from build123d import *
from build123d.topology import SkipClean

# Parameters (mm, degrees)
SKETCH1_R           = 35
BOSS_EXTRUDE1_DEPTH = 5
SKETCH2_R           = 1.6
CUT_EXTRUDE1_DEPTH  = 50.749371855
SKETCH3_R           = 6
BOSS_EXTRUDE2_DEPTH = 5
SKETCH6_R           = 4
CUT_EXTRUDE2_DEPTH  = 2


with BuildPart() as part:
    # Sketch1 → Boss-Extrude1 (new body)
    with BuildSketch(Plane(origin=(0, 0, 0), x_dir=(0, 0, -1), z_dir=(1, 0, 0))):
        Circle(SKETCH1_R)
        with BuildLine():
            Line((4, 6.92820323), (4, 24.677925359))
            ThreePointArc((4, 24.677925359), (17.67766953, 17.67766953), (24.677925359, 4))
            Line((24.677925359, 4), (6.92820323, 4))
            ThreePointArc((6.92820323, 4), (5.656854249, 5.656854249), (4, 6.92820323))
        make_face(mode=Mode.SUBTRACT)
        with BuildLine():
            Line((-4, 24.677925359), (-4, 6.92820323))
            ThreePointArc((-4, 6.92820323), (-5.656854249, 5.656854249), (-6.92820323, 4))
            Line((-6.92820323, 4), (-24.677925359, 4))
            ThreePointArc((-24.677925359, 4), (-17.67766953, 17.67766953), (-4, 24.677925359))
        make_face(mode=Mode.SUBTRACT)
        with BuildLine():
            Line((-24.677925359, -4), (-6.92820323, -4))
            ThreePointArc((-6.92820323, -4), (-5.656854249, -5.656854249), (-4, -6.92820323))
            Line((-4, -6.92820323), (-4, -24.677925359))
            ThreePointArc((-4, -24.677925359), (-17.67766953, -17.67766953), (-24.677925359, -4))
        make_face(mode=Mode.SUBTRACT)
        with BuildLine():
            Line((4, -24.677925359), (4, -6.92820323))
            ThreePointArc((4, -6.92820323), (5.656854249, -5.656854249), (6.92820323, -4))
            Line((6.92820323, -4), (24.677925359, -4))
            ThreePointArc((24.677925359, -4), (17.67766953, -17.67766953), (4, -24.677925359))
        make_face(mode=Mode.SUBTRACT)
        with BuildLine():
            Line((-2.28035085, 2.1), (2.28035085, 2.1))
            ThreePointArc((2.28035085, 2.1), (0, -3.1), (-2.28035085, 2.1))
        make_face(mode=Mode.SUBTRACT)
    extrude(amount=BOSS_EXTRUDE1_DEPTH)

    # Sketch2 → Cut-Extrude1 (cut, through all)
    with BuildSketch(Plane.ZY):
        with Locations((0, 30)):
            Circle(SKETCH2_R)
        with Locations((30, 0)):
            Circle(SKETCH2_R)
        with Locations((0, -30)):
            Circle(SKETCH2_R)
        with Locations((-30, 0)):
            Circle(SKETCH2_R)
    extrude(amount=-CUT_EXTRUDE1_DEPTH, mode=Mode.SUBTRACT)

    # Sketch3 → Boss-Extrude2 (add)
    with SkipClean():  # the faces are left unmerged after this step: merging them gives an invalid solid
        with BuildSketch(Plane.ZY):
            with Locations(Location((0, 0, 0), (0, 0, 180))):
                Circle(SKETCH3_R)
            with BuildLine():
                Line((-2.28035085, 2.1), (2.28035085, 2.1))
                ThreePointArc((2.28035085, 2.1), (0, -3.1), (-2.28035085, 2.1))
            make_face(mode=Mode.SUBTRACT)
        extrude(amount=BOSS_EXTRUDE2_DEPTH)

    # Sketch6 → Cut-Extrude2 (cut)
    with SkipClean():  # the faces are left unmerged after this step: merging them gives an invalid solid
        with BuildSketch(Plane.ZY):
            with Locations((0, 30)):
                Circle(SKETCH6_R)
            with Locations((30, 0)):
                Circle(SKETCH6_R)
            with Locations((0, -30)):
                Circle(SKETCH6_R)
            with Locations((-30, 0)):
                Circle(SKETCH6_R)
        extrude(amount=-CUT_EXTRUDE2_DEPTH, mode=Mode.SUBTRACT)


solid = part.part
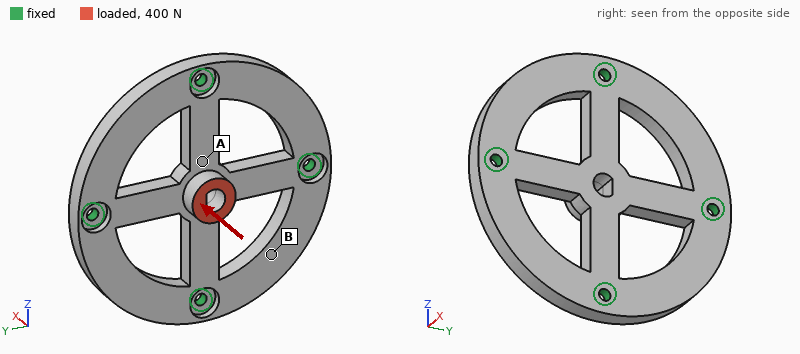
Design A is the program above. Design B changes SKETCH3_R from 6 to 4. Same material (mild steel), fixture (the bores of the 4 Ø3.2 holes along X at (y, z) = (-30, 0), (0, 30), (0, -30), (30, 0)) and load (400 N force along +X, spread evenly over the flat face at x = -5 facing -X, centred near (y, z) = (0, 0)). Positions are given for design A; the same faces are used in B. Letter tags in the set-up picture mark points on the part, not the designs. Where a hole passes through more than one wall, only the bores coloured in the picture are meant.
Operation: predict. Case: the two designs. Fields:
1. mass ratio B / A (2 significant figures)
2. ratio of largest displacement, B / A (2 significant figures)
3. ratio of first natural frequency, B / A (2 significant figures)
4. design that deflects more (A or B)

0.98
1.2
1.0
B
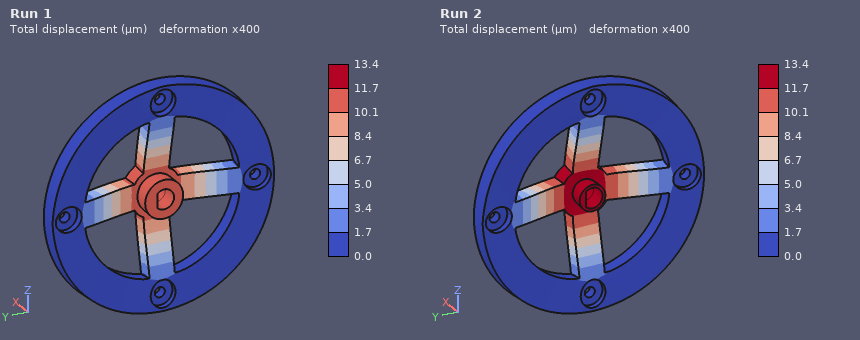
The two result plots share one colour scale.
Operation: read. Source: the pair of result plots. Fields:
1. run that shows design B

Run 2
